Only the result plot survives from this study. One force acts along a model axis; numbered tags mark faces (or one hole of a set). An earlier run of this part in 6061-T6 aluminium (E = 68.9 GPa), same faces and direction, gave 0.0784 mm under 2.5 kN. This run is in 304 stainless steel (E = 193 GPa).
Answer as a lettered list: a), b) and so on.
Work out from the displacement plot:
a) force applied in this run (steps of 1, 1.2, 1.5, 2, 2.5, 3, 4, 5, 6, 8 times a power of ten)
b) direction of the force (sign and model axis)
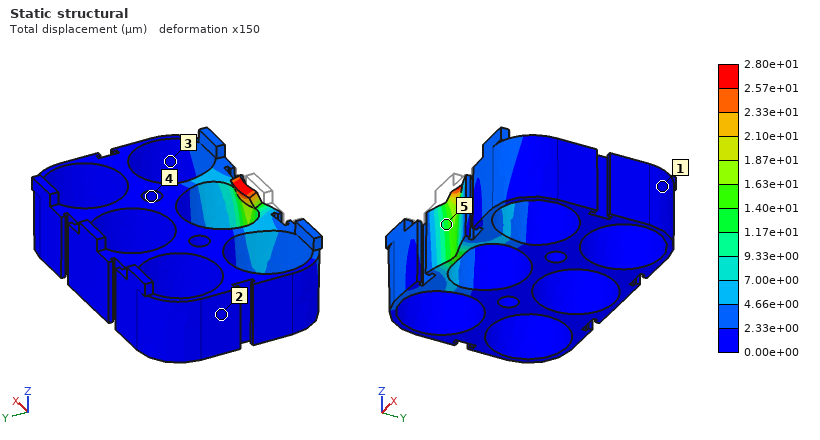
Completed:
a) 2.5 kN
b) +Y
